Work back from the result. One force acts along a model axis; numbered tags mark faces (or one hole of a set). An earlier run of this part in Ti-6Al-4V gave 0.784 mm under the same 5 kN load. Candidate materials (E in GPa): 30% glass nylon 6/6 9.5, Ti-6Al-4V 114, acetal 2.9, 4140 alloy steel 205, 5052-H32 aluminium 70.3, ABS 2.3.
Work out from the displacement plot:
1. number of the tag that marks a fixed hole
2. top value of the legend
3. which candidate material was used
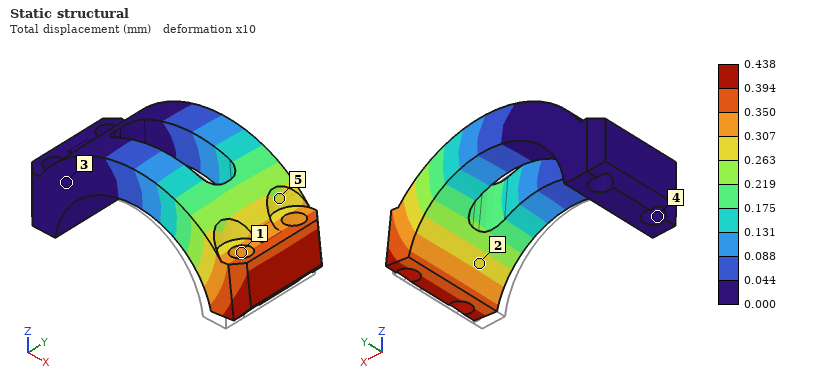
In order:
4
0.438 mm
4140 alloy steel
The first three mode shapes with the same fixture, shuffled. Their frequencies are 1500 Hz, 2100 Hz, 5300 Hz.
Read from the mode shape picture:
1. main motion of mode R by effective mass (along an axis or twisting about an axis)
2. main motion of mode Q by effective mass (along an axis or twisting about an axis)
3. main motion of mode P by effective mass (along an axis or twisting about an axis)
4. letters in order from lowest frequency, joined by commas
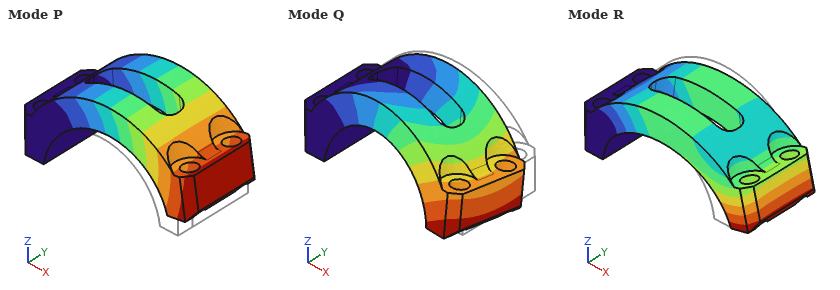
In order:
along X
along Y
along Z
P, Q, R
